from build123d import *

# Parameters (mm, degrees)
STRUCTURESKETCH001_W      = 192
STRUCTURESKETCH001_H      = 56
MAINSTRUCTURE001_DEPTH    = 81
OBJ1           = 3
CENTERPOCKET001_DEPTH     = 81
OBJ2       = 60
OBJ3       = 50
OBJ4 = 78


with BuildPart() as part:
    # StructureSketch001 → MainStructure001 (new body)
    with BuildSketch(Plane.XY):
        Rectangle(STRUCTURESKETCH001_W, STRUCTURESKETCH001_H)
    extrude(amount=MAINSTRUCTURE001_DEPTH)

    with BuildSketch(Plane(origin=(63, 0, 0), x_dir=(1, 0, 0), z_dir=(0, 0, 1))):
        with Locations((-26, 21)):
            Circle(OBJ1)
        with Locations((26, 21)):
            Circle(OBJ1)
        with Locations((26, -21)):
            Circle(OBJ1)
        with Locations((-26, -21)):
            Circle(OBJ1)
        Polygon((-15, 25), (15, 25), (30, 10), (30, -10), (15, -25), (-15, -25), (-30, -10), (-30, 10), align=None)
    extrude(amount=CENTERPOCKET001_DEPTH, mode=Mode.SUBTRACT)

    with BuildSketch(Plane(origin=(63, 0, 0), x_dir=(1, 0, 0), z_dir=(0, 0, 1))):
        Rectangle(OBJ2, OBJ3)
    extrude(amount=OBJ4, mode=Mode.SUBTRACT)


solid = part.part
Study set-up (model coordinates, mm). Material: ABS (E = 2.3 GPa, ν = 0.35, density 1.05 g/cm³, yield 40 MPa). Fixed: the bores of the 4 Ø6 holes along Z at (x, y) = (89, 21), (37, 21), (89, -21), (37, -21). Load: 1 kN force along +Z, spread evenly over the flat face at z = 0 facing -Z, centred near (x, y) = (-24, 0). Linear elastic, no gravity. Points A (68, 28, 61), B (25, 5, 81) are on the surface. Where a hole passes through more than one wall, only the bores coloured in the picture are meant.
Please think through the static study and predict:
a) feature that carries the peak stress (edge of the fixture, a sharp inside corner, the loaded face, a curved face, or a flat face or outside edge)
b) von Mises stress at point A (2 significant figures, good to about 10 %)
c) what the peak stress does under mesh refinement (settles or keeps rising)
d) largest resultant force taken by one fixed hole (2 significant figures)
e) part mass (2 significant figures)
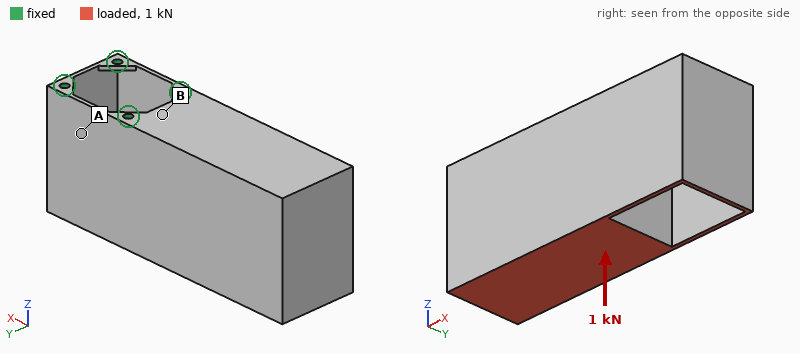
edge of the fixture
6.6 MPa
keeps rising
1.0 kN
660 g
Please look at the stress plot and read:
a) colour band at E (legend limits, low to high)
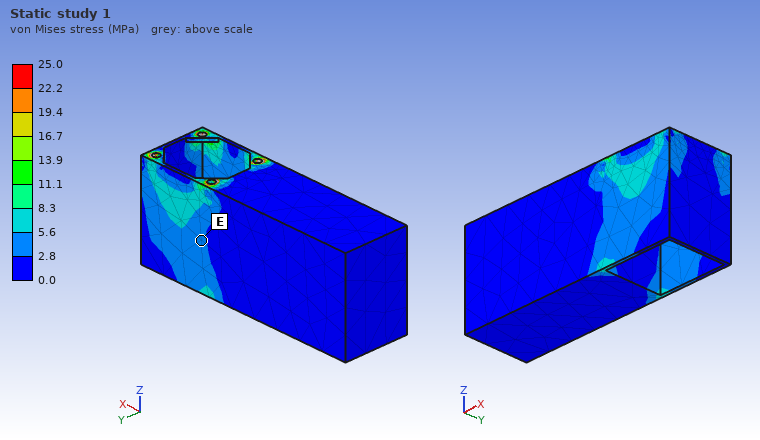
2.8 to 5.6 MPa
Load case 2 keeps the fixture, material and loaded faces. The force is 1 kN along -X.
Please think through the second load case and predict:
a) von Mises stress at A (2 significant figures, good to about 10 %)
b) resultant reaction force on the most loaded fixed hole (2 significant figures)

8.6 MPa
760 N
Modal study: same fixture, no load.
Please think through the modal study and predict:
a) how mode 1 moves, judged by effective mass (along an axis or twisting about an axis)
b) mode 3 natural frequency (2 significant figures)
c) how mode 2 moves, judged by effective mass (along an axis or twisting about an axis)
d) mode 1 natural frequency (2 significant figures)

along Z
440 Hz
along Y
180 Hz
